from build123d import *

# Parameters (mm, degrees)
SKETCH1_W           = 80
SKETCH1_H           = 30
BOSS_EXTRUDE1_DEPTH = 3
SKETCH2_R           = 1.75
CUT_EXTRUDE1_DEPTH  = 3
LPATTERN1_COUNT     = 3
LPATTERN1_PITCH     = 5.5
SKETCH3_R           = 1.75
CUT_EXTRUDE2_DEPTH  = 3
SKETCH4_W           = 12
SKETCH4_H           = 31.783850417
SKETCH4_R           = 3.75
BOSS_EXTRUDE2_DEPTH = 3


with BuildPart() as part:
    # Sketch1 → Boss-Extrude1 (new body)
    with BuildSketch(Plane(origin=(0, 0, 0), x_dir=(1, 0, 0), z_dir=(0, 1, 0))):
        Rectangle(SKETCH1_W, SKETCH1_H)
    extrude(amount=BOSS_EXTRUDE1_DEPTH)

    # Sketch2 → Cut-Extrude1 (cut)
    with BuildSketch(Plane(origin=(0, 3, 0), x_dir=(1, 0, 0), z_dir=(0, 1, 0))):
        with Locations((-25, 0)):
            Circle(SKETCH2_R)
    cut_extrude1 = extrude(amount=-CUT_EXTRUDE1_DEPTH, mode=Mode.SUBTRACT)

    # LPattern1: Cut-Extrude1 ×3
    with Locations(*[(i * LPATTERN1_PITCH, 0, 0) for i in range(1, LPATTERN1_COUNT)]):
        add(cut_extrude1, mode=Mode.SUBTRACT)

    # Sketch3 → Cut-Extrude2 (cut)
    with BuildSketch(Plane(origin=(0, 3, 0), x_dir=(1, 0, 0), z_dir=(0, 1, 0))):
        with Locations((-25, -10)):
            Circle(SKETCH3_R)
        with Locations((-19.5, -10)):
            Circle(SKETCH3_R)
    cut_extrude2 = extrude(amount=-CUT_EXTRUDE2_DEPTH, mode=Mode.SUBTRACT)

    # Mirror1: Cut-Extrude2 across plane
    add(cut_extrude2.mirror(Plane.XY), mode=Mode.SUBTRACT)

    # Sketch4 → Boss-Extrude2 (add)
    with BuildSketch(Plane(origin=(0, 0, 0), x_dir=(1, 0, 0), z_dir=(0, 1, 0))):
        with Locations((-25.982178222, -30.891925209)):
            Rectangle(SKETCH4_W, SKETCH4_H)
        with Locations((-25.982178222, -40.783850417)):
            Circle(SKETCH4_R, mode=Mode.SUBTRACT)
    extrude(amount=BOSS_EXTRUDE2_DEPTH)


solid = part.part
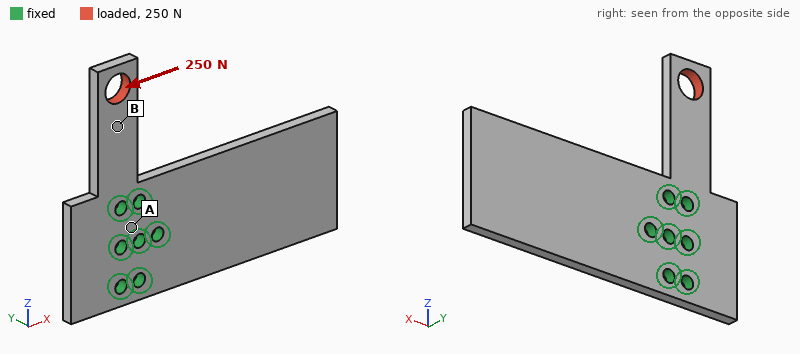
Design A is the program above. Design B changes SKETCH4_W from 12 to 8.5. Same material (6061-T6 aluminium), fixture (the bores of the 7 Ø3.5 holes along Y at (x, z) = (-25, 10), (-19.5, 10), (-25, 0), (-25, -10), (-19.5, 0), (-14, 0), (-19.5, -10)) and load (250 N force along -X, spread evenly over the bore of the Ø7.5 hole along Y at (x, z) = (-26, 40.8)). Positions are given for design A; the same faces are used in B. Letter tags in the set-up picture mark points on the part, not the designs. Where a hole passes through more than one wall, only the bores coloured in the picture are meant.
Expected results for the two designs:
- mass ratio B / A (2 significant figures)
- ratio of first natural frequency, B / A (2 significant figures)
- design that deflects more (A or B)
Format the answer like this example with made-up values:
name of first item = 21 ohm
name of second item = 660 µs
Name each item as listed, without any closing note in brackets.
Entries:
mass ratio B / A = 0.96
ratio of first natural frequency, B / A = 1.00
design that deflects more = B
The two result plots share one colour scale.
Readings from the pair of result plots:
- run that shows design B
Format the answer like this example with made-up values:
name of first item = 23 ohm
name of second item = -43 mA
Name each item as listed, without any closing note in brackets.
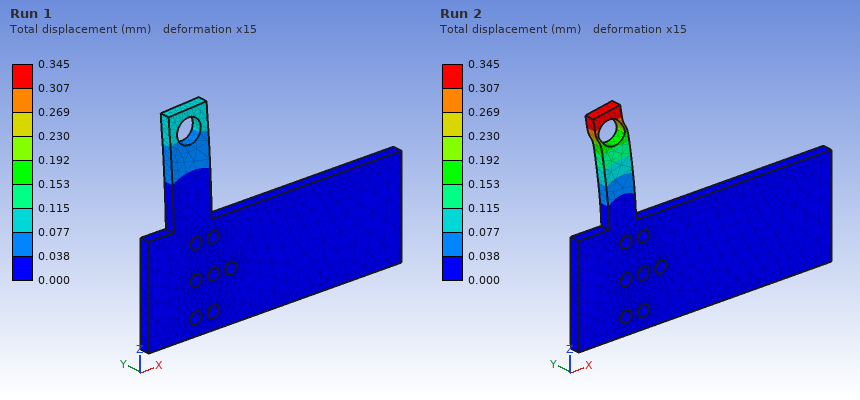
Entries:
run that shows design B = Run 2
